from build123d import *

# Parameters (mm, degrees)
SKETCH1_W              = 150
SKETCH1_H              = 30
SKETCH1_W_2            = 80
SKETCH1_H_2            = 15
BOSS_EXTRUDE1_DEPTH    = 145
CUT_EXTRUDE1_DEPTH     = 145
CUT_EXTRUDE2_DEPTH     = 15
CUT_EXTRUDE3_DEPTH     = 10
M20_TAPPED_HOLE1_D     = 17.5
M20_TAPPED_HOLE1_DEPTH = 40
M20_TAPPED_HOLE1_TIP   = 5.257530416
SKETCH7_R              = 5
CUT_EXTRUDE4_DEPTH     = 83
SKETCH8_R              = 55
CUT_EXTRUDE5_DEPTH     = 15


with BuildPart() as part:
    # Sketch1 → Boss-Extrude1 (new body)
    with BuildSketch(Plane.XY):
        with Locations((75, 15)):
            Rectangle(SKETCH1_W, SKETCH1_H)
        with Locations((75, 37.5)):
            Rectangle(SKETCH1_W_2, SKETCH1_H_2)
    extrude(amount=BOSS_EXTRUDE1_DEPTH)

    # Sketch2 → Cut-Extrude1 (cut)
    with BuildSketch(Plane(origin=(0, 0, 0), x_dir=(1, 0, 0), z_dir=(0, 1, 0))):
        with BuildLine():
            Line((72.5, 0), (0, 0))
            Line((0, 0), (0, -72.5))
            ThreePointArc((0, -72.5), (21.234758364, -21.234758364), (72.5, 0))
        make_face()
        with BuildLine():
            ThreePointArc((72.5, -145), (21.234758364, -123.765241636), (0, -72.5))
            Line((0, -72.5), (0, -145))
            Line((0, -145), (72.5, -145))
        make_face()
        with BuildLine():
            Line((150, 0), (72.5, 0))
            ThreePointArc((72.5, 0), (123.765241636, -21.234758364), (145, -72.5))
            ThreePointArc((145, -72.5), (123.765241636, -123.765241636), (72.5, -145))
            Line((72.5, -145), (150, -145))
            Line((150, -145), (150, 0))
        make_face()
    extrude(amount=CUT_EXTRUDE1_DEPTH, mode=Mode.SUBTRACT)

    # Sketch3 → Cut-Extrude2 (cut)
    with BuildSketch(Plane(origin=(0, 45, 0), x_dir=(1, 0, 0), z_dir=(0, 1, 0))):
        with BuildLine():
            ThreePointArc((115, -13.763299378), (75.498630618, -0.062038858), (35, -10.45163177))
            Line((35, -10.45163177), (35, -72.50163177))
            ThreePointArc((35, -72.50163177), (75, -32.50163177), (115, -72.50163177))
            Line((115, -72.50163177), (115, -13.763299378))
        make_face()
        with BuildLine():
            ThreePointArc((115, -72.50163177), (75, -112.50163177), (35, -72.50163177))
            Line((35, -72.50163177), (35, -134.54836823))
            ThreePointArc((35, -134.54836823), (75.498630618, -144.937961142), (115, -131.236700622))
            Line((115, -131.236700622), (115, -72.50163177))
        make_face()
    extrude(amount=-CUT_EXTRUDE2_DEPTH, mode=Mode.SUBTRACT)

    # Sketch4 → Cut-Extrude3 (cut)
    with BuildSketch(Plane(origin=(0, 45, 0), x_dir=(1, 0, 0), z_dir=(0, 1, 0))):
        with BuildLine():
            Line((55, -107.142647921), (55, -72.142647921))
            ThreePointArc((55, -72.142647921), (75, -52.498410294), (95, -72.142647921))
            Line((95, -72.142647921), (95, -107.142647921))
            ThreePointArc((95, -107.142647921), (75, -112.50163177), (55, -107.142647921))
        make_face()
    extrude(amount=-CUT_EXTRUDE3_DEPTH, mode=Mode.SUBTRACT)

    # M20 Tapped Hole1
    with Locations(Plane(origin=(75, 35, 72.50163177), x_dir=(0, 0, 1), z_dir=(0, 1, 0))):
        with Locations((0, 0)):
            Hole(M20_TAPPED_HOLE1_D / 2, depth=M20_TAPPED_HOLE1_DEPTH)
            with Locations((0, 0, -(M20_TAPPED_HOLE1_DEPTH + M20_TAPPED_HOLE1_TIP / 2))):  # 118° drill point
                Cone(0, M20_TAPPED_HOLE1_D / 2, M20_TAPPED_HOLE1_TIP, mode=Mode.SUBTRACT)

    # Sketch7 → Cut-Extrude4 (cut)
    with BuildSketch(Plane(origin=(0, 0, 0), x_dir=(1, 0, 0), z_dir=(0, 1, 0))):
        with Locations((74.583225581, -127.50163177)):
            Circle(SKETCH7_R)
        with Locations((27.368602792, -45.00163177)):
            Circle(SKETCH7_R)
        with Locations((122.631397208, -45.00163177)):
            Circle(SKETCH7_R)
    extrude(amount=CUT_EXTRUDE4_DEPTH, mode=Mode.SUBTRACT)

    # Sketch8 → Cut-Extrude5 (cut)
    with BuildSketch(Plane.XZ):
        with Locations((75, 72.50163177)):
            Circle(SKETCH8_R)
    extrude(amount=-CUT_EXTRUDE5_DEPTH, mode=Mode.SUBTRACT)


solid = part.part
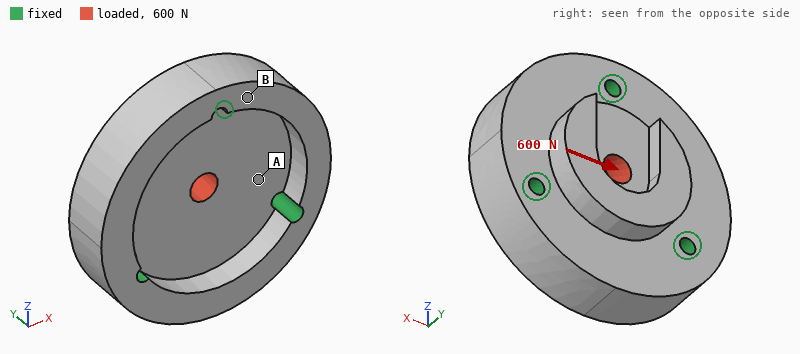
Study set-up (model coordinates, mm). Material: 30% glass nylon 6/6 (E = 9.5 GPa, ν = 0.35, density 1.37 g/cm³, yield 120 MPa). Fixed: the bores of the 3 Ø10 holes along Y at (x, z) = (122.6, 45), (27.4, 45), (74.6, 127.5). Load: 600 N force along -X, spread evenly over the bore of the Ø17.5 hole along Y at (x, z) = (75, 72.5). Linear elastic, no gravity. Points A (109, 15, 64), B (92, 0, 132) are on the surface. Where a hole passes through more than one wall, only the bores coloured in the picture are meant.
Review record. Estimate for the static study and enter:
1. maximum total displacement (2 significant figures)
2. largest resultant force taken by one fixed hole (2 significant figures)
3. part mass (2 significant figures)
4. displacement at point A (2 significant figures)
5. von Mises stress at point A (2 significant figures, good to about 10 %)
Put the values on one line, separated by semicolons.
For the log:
2.6 µm; 220 N; 540 g; 1.2 µm; 0.32 MPa
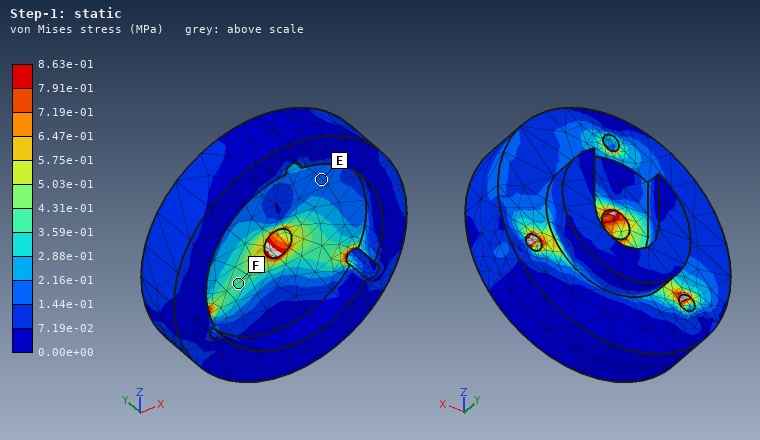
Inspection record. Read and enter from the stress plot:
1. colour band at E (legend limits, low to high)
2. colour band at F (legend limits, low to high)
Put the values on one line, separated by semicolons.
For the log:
1.44e-01 to 2.16e-01 MPa; 3.59e-01 to 4.31e-01 MPa
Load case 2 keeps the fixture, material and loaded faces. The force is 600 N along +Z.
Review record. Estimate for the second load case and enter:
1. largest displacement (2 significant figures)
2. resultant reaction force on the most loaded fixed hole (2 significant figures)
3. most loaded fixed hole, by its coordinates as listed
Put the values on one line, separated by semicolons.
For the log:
2.7 µm; 220 N; (74.6, 127.5)
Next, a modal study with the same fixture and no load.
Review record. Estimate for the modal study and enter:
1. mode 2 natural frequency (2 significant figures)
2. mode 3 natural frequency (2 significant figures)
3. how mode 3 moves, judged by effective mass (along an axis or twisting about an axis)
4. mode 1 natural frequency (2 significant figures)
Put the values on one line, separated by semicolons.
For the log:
3400 Hz; 3500 Hz; along Y; 3200 Hz
